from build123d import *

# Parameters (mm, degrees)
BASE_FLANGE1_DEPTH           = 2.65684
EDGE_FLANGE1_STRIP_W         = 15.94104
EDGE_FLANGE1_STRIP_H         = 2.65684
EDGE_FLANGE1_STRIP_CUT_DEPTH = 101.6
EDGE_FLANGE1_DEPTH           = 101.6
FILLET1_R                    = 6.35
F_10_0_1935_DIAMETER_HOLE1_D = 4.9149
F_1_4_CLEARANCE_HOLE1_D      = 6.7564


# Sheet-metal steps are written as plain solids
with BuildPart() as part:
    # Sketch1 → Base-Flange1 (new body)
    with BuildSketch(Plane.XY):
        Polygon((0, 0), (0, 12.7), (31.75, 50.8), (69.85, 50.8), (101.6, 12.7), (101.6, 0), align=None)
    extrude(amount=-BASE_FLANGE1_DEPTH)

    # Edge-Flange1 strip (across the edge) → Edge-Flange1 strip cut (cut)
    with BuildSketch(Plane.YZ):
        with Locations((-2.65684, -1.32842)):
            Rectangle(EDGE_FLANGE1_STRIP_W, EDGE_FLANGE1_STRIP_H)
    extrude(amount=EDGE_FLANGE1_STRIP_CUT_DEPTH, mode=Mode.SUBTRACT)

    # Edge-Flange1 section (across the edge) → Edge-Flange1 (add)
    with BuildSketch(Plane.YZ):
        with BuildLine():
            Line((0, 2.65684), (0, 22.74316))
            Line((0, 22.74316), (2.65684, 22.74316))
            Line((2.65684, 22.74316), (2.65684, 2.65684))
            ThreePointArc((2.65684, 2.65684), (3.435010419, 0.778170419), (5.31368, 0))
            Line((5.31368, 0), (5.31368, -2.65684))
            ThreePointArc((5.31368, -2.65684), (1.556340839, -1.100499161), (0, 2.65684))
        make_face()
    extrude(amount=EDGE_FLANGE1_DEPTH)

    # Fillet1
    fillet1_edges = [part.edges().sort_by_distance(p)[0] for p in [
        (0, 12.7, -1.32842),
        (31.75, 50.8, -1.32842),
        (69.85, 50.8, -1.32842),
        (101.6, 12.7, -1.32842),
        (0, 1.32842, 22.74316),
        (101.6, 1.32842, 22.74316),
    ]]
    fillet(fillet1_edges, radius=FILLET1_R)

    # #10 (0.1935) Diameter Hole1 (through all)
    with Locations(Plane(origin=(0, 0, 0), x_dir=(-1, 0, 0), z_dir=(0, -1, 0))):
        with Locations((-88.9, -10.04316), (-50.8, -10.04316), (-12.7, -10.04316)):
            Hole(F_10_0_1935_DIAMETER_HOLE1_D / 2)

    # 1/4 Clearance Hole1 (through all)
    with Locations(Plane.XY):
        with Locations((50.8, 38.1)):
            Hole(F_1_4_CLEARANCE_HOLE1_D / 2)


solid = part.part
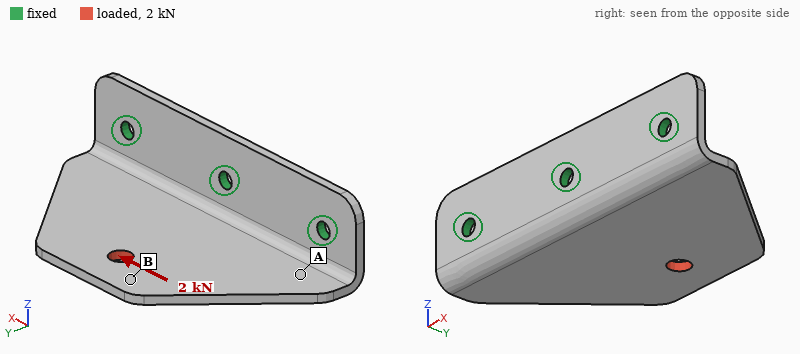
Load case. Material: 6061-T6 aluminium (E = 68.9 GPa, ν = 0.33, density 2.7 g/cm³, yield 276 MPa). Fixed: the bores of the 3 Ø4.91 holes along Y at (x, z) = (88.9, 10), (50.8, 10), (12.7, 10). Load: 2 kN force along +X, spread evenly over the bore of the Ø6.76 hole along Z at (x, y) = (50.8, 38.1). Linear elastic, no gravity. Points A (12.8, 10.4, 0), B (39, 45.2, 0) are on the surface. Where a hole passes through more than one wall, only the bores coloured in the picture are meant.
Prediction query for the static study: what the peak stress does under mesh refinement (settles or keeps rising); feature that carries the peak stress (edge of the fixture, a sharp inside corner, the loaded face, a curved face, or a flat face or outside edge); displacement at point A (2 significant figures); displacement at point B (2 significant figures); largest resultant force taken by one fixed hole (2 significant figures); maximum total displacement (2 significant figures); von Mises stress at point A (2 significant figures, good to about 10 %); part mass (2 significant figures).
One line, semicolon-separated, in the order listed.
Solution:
keeps rising; edge of the fixture; 0.15 mm; 0.19 mm; 1.2 kN; 0.28 mm; 61 MPa; 43 g
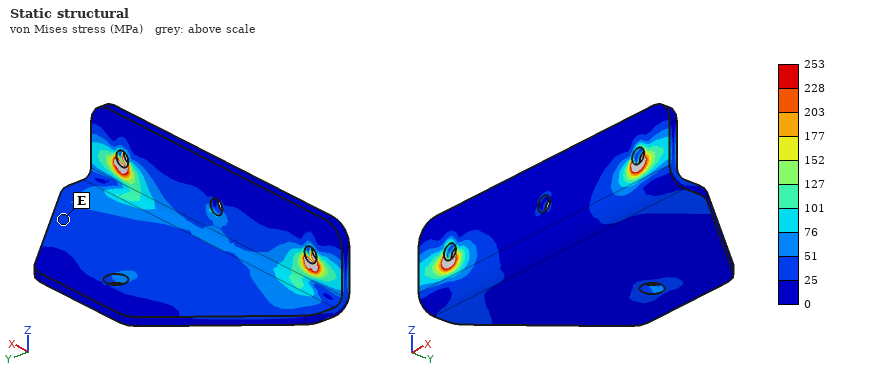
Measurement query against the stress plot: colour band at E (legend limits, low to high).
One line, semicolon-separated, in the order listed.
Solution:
25 to 51 MPa
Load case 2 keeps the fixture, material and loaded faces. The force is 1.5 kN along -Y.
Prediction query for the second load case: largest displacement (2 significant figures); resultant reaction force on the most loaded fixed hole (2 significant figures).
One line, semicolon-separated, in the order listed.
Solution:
0.47 mm; 570 N
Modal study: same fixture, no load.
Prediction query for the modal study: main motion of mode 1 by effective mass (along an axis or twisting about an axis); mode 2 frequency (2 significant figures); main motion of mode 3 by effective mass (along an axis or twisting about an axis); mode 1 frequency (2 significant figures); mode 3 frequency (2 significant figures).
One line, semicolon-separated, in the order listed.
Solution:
along Z; 2000 Hz; along Y; 880 Hz; 3700 Hz
